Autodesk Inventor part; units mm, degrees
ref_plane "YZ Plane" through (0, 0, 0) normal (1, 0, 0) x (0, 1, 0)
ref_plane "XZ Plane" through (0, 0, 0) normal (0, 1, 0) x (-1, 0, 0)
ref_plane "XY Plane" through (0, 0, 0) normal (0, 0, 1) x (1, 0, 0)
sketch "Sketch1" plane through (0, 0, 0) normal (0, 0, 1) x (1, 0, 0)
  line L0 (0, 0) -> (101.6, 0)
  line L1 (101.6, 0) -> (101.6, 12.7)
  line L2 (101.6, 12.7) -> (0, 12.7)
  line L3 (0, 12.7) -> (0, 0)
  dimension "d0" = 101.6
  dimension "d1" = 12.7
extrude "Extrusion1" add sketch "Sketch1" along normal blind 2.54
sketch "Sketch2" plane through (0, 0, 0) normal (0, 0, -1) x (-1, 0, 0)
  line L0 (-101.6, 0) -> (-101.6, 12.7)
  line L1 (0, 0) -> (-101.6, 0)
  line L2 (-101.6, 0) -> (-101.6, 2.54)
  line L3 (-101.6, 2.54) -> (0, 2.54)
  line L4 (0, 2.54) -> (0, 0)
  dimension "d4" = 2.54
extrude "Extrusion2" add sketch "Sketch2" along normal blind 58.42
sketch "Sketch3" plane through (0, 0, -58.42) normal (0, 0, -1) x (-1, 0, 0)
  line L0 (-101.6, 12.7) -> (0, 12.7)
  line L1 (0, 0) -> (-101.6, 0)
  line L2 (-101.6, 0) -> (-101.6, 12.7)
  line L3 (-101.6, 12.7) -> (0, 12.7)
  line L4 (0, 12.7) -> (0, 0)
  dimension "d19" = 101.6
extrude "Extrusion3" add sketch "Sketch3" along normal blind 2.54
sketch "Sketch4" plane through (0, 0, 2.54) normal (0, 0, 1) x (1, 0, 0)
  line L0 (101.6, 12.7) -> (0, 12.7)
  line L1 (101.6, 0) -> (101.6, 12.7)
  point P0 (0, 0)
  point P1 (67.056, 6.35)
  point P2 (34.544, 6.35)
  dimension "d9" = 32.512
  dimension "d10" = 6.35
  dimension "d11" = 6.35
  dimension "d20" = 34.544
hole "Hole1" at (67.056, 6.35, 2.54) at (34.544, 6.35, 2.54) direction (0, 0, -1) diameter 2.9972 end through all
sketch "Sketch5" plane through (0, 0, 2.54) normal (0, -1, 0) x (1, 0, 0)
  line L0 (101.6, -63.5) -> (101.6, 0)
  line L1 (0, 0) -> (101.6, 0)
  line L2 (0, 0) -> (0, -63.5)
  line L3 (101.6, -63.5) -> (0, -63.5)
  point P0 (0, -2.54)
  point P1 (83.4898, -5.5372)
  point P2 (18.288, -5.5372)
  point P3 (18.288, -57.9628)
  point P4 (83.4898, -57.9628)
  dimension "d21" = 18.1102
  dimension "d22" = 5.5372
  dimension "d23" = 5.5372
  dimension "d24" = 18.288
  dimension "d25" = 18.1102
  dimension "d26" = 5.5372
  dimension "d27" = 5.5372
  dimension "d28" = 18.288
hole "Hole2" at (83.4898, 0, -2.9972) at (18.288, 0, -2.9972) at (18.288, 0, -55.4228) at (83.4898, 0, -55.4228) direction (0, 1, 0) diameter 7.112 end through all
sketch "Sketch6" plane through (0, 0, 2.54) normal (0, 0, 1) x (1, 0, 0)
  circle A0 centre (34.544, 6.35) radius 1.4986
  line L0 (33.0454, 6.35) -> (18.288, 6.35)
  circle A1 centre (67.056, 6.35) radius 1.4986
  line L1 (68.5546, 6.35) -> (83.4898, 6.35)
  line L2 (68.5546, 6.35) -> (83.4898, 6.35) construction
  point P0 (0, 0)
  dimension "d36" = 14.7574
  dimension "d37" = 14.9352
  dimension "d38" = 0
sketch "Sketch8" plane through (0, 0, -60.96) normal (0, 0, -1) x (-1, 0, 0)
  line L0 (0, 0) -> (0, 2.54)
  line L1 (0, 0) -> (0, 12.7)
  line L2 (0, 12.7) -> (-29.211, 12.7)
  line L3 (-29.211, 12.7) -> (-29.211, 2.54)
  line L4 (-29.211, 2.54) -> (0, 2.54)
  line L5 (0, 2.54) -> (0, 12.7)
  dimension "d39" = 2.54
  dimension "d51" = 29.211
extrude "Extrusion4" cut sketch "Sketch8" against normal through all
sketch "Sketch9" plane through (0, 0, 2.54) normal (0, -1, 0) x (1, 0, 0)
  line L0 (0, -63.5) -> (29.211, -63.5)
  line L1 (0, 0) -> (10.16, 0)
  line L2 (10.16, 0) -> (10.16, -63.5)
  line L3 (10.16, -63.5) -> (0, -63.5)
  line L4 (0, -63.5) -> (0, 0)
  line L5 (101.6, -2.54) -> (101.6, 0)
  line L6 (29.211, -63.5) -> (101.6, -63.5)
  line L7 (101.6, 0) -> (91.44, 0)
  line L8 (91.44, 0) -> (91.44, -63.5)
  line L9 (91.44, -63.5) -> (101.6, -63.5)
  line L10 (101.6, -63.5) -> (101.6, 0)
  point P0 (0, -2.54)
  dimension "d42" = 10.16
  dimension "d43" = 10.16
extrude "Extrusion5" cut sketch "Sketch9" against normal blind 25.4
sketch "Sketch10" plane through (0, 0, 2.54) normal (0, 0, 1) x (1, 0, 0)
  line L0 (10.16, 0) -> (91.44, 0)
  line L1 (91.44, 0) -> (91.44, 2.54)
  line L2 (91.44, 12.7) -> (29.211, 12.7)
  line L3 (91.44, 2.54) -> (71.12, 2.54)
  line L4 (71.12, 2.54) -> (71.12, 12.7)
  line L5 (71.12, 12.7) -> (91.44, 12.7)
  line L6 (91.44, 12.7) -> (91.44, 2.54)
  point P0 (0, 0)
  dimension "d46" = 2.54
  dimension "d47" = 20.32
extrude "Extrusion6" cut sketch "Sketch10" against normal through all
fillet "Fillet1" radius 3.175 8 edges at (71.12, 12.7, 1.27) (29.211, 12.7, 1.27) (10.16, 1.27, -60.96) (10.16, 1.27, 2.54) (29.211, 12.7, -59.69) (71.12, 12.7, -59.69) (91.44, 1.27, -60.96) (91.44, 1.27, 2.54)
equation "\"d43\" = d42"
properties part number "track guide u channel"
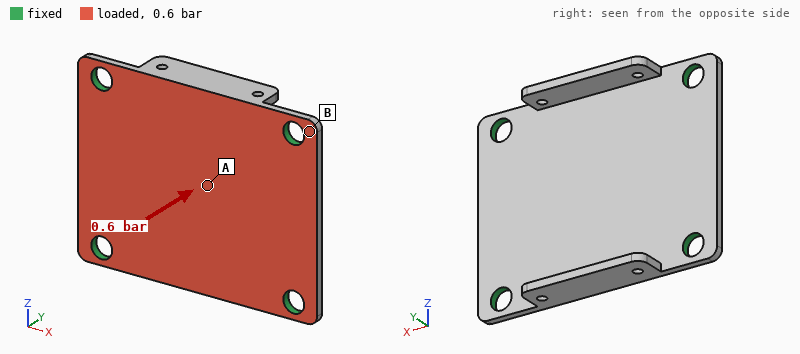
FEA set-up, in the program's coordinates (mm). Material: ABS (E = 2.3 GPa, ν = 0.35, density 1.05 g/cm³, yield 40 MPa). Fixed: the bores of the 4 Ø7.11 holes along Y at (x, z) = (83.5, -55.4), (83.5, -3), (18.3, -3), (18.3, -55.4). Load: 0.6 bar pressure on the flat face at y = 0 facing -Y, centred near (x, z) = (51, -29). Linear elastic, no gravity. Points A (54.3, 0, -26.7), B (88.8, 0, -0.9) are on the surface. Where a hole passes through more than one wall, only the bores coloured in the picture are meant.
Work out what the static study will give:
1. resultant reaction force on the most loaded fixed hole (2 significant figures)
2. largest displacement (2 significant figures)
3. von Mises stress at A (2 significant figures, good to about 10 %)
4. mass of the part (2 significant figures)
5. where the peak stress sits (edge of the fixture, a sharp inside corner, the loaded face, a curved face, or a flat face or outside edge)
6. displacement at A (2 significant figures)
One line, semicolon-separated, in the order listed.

77 N; 0.91 mm; 8.6 MPa; 15 g; the loaded face; 0.89 mm
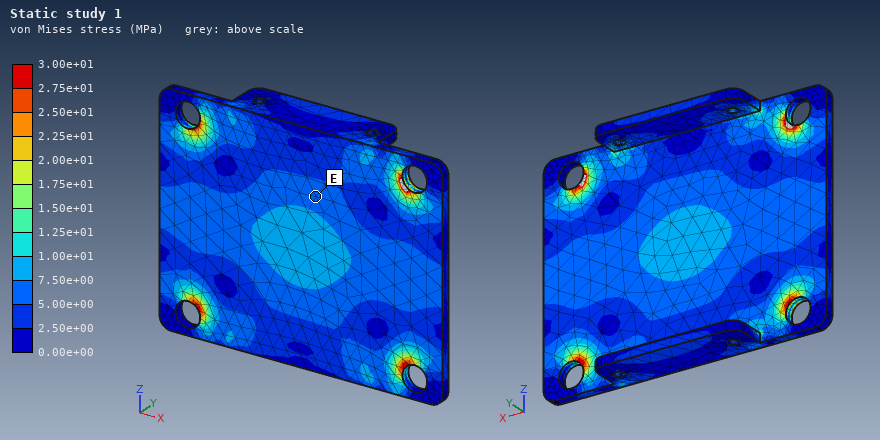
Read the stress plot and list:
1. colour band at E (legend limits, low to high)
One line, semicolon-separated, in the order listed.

5.00e+00 to 7.50e+00 MPa
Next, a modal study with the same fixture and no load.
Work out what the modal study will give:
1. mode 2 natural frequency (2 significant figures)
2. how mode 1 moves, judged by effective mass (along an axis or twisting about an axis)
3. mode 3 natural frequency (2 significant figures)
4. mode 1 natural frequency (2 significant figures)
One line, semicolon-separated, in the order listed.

1700 Hz; along Y; 1700 Hz; 960 Hz
